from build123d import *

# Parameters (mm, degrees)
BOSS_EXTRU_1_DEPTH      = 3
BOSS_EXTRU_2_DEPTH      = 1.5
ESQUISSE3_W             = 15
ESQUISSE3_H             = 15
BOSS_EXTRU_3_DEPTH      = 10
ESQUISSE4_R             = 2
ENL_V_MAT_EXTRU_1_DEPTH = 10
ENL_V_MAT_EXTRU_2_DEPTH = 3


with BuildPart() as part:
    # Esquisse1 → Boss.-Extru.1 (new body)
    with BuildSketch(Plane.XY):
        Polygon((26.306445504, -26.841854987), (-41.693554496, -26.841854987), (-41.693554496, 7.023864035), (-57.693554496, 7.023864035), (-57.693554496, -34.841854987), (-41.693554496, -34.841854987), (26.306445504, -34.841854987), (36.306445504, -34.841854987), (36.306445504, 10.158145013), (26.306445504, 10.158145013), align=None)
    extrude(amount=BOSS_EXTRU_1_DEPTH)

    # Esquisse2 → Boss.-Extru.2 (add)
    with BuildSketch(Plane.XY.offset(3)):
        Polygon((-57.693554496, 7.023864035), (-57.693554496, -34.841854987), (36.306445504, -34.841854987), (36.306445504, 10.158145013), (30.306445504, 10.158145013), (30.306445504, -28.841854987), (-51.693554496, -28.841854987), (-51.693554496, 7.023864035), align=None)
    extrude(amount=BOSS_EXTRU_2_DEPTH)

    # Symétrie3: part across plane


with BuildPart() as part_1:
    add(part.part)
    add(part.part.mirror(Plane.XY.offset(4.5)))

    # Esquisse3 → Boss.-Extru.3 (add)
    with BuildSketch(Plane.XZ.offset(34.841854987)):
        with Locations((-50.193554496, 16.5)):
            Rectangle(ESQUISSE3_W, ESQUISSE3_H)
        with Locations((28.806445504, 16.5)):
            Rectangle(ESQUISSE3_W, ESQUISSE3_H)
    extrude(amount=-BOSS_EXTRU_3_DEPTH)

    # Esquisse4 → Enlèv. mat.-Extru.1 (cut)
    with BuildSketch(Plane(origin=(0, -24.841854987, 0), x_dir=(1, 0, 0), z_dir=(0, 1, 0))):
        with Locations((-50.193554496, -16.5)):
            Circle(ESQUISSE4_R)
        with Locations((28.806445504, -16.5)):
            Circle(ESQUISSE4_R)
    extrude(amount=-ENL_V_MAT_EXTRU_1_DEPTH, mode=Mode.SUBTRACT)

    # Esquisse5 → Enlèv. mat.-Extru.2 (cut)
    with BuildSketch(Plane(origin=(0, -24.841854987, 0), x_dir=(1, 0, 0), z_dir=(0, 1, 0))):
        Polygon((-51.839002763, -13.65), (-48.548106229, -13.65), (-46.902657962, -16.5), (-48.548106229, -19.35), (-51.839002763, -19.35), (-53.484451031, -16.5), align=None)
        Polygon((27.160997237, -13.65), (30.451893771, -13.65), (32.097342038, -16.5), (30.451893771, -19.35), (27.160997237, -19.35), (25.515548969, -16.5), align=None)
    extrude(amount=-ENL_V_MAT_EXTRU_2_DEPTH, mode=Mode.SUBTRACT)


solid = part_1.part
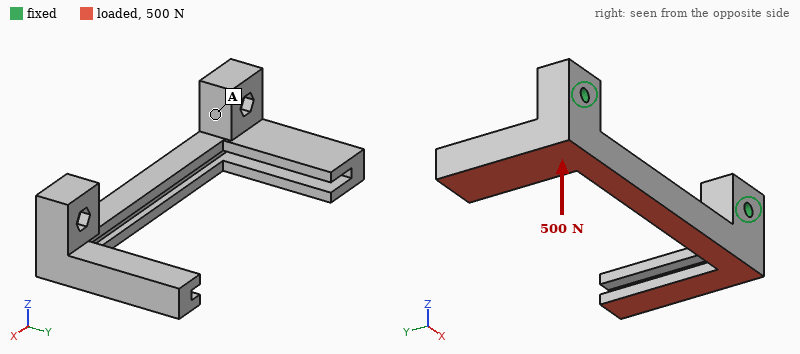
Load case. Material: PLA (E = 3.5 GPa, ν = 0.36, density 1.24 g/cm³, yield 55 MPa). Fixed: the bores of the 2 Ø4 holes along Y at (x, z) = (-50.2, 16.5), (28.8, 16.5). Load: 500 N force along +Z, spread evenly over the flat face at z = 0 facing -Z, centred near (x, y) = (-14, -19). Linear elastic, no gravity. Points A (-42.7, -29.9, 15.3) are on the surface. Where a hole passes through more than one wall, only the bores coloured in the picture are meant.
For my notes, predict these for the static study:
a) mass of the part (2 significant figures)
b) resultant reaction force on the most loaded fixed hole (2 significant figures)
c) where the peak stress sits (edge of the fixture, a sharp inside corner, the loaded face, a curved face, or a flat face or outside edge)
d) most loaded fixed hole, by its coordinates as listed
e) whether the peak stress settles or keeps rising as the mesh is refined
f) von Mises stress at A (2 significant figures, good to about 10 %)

21 g
280 N
edge of the fixture
(-50.2, 16.5)
keeps rising
4.5 MPa
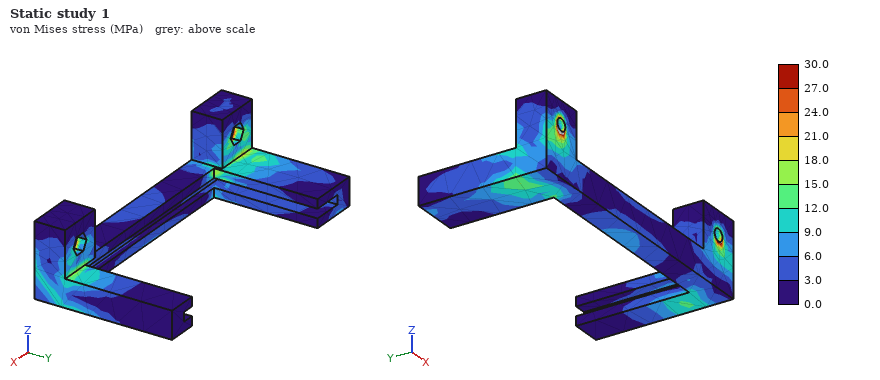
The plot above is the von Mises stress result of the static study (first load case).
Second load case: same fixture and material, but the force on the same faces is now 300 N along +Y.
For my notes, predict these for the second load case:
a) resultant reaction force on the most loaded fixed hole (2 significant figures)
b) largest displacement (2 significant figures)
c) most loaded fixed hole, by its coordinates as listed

170 N
0.42 mm
(-50.2, 16.5)
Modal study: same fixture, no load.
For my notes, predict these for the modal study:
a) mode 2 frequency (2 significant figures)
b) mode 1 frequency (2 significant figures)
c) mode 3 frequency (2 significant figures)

1200 Hz
1100 Hz
1200 Hz
